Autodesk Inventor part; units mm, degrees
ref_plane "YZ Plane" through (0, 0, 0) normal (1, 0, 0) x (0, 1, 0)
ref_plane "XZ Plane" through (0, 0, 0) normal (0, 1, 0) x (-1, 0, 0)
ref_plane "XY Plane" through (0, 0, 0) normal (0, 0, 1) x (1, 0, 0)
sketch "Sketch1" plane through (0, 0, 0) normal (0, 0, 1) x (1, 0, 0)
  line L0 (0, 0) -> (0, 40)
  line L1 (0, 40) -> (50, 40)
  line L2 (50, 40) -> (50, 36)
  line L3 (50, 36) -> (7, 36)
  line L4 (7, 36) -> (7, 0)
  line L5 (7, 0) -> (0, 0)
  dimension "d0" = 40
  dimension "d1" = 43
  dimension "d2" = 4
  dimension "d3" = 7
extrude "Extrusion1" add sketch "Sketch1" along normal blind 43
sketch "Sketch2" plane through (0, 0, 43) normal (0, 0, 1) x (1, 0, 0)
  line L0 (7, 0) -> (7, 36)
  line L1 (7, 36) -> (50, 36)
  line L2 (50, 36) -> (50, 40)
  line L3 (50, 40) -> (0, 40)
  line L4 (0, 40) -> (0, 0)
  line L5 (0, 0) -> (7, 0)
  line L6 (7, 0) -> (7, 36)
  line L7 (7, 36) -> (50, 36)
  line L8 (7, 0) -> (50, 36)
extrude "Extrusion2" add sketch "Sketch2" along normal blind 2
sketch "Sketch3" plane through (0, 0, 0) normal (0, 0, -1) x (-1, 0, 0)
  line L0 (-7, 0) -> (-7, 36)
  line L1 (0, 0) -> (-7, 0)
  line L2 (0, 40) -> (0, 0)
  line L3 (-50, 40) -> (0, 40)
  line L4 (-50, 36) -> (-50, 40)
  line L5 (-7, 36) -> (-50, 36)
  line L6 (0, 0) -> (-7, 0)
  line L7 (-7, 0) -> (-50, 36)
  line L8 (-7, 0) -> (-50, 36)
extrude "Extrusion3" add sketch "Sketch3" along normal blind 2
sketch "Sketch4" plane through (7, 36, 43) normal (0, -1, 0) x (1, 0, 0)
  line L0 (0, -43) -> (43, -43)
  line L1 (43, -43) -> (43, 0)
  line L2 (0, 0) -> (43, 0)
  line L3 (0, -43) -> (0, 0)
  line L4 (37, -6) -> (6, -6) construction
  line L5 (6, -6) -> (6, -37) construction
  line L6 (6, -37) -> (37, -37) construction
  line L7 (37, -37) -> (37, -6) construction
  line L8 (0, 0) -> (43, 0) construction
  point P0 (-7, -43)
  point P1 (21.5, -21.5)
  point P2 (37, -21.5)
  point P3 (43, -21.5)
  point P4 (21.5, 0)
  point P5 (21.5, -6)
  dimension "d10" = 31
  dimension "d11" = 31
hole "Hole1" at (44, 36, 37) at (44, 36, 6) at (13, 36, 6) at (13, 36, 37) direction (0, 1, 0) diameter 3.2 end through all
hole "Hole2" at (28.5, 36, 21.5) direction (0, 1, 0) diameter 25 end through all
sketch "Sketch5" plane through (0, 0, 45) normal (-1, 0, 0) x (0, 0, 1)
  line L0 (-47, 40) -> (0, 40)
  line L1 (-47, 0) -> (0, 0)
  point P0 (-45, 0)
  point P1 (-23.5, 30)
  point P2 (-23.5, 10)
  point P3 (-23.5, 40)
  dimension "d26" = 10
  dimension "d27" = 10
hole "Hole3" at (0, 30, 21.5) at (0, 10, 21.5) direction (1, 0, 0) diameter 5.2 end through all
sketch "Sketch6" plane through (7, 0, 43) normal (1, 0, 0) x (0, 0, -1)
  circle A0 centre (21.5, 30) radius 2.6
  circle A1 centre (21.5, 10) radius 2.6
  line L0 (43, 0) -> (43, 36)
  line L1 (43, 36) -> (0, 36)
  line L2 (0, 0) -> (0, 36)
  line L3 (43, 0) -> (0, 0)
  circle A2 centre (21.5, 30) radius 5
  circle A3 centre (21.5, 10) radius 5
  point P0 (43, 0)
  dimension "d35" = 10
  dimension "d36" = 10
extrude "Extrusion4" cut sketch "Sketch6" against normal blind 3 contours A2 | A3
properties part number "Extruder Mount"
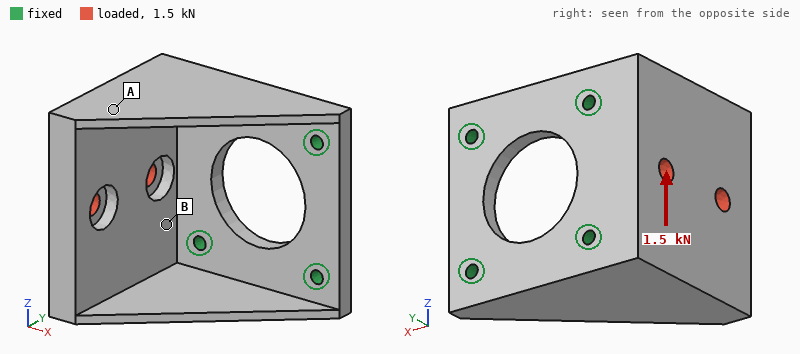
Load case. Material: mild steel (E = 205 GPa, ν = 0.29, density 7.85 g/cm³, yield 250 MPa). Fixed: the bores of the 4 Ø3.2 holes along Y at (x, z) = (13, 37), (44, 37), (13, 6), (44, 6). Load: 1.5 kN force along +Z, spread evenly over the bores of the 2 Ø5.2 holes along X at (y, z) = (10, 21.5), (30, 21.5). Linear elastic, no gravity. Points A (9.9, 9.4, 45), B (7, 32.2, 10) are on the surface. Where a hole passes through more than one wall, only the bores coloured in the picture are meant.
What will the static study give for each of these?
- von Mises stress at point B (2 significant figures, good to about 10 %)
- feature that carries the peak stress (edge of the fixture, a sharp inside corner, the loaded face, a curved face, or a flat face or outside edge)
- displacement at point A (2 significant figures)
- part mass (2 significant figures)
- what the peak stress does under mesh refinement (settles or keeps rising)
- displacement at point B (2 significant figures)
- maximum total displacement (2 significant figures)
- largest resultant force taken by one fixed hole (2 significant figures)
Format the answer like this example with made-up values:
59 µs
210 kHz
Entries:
22 MPa
edge of the fixture
12 µm
170 g
keeps rising
3.5 µm
14 µm
1.2 kN
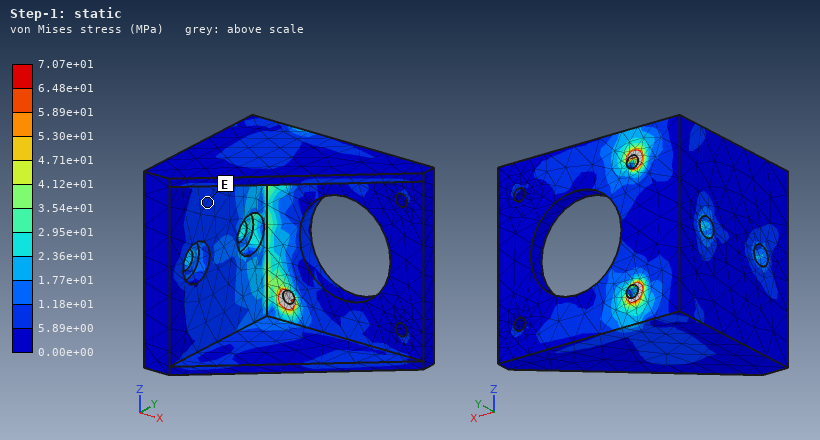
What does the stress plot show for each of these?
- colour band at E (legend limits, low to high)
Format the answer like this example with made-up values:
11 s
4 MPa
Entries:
5.89e+00 to 1.18e+01 MPa
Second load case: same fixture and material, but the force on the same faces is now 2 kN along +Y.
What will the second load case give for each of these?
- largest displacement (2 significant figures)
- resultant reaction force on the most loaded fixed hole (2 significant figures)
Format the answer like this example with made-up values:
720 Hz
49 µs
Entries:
18 µm
1.3 kN
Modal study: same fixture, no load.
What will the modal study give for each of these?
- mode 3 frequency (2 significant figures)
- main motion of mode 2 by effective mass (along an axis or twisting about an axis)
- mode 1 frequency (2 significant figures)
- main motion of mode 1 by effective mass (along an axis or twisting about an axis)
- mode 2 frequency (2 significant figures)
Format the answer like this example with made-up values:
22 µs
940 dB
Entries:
7700 Hz
along Z
4800 Hz
along X
5300 Hz
